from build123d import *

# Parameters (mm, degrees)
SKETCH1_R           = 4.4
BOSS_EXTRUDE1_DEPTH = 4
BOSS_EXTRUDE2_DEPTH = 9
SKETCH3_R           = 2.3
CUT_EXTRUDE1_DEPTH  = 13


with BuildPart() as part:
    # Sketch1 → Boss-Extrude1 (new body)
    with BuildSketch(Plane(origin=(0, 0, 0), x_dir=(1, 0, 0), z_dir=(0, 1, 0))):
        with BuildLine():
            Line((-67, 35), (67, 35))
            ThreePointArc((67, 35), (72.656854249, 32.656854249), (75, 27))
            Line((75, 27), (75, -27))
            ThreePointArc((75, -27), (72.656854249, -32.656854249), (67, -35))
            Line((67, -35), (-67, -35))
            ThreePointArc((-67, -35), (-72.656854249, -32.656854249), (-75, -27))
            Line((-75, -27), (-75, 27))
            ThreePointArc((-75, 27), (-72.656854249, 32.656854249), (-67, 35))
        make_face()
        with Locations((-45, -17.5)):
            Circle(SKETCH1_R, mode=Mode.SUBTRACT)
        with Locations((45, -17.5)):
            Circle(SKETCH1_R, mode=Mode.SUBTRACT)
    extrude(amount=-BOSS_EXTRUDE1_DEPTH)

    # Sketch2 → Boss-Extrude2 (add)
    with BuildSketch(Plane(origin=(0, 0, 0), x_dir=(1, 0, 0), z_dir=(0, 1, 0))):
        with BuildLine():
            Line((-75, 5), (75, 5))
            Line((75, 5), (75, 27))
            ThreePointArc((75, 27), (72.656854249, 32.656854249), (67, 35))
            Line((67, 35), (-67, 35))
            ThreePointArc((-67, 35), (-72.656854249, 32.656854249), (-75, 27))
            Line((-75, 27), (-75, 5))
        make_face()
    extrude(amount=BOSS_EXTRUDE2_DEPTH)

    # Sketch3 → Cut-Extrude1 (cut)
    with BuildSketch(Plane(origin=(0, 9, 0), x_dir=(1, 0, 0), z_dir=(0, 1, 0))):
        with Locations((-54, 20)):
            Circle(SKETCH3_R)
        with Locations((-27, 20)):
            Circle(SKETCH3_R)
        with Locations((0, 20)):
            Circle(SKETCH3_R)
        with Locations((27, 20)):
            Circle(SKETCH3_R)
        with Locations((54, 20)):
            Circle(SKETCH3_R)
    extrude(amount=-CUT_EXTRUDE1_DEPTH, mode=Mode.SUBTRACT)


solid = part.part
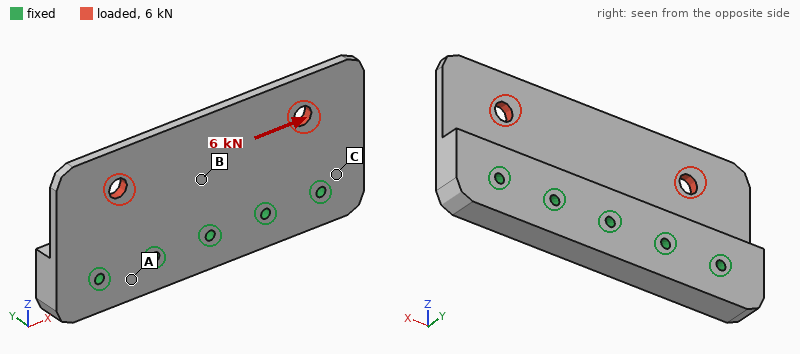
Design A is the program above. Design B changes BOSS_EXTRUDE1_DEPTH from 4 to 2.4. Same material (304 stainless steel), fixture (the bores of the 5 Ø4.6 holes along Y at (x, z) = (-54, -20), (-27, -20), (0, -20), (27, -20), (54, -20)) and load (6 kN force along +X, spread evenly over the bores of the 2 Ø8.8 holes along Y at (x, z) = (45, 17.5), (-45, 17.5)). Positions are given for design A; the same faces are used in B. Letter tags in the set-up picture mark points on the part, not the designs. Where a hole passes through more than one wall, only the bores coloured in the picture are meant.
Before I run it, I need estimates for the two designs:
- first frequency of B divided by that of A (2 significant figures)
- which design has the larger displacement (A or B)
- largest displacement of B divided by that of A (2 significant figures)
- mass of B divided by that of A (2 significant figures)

0.64
B
1.6
0.80
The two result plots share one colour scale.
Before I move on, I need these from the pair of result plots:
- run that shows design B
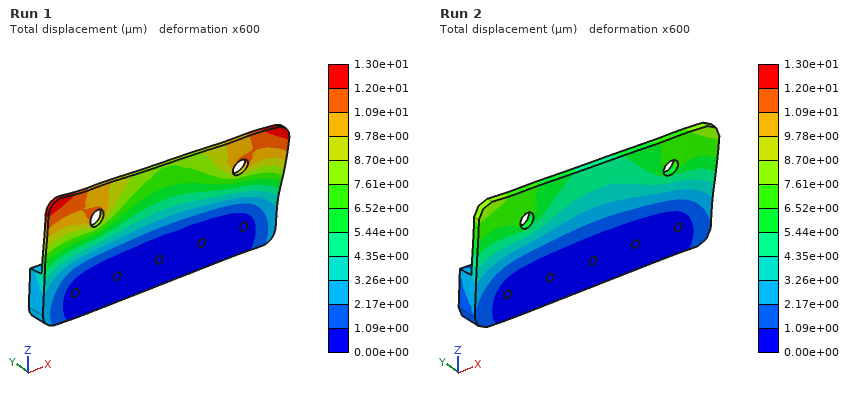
Run 1
